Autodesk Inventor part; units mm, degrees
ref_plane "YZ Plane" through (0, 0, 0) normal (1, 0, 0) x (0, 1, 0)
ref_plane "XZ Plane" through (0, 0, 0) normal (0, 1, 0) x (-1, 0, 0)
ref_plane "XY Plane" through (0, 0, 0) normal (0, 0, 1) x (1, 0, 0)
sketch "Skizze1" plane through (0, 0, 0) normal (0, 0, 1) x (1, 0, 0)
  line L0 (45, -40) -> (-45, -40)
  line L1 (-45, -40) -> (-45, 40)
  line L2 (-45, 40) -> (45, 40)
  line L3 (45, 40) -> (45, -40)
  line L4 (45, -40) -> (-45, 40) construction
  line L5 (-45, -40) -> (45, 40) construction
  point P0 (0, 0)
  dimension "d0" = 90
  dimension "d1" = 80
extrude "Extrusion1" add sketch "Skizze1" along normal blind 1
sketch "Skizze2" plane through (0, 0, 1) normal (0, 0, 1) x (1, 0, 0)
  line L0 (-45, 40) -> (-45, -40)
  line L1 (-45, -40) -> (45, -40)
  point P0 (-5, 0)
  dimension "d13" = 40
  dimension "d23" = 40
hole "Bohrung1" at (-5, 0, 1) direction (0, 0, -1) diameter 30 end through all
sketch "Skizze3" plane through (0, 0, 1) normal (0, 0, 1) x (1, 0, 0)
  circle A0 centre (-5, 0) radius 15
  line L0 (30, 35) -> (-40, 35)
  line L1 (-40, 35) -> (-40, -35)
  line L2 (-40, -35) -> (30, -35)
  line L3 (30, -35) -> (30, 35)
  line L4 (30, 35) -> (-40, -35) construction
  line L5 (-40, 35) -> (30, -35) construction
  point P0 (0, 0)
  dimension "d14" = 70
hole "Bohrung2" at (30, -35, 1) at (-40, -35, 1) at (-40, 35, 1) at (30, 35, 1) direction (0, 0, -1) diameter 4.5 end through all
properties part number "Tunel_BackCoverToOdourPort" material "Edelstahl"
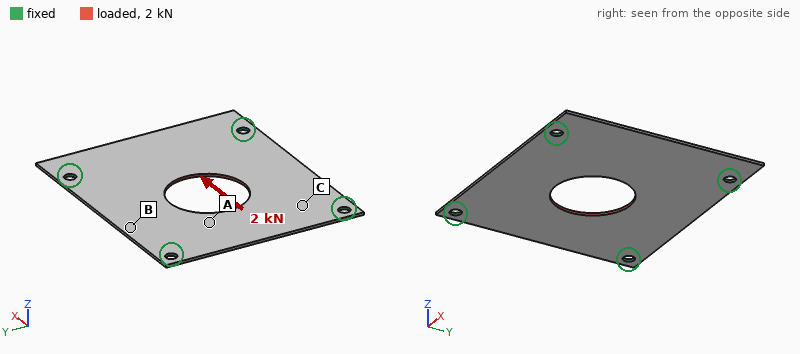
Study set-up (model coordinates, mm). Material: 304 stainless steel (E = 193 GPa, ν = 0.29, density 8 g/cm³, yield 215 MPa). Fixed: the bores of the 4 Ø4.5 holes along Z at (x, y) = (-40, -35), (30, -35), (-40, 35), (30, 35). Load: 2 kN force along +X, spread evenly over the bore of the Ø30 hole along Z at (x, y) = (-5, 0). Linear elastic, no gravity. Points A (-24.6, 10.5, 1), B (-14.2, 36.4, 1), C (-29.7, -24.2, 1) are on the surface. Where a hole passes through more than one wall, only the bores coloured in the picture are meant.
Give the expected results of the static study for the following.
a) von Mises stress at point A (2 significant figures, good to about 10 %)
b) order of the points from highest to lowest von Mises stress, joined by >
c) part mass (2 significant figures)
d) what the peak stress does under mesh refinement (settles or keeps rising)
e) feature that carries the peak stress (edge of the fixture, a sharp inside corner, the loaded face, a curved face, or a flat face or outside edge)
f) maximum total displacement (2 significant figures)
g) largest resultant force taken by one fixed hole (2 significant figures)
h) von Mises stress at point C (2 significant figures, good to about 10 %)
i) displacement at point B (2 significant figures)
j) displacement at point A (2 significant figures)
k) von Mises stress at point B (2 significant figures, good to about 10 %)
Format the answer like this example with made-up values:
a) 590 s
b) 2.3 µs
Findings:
a) 21 MPa
b) C > A > B
c) 51 g
d) keeps rising
e) edge of the fixture
f) 8.2 µm
g) 550 N
h) 26 MPa
i) 2.8 µm
j) 6.5 µm
k) 11 MPa
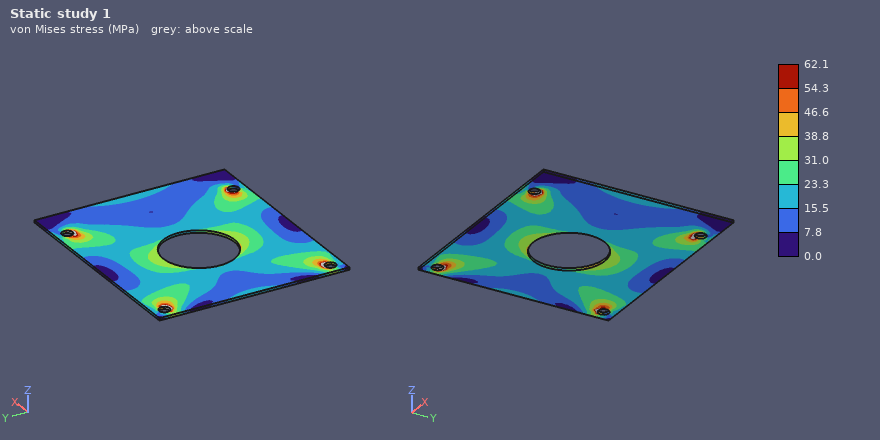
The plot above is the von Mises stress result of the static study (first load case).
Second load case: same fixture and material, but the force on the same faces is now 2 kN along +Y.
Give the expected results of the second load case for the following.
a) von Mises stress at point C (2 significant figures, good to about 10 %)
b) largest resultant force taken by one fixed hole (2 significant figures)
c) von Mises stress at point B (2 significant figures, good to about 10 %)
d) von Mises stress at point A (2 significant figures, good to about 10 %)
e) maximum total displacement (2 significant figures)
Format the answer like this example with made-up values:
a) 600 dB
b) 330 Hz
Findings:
a) 27 MPa
b) 570 N
c) 12 MPa
d) 25 MPa
e) 8.1 µm
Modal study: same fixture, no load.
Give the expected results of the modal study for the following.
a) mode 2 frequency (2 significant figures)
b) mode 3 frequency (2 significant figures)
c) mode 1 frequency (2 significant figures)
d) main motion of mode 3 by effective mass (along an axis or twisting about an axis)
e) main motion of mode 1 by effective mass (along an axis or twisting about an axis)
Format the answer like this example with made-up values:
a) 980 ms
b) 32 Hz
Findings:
a) 1100 Hz
b) 1200 Hz
c) 760 Hz
d) twisting about X
e) along Z
